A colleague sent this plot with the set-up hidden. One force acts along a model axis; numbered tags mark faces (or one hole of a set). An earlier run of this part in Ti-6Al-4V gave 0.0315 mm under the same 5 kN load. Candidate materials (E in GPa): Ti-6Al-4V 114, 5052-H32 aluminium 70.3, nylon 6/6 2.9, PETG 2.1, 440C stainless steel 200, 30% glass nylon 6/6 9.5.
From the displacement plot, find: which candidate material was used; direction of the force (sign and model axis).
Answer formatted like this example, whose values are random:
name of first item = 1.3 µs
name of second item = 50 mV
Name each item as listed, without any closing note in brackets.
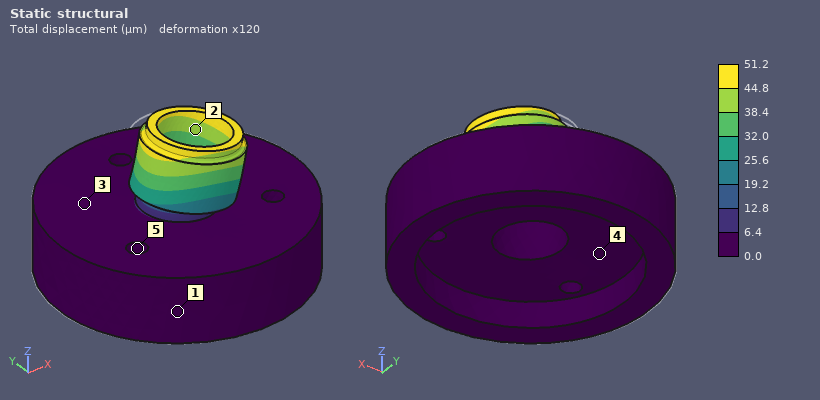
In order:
which candidate material was used = 5052-H32 aluminium
direction of the force = +X
